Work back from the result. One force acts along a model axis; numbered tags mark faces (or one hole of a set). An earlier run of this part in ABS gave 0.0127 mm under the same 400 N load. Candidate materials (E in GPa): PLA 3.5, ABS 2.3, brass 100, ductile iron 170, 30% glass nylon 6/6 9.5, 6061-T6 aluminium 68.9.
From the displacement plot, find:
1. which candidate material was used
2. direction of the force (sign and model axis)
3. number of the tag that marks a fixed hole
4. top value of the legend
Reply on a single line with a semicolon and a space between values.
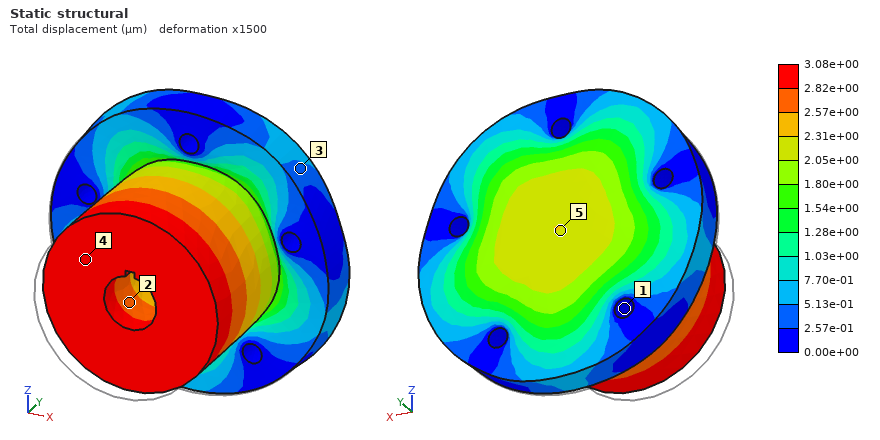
30% glass nylon 6/6; +Y; 1; 3.08e+00 µm
